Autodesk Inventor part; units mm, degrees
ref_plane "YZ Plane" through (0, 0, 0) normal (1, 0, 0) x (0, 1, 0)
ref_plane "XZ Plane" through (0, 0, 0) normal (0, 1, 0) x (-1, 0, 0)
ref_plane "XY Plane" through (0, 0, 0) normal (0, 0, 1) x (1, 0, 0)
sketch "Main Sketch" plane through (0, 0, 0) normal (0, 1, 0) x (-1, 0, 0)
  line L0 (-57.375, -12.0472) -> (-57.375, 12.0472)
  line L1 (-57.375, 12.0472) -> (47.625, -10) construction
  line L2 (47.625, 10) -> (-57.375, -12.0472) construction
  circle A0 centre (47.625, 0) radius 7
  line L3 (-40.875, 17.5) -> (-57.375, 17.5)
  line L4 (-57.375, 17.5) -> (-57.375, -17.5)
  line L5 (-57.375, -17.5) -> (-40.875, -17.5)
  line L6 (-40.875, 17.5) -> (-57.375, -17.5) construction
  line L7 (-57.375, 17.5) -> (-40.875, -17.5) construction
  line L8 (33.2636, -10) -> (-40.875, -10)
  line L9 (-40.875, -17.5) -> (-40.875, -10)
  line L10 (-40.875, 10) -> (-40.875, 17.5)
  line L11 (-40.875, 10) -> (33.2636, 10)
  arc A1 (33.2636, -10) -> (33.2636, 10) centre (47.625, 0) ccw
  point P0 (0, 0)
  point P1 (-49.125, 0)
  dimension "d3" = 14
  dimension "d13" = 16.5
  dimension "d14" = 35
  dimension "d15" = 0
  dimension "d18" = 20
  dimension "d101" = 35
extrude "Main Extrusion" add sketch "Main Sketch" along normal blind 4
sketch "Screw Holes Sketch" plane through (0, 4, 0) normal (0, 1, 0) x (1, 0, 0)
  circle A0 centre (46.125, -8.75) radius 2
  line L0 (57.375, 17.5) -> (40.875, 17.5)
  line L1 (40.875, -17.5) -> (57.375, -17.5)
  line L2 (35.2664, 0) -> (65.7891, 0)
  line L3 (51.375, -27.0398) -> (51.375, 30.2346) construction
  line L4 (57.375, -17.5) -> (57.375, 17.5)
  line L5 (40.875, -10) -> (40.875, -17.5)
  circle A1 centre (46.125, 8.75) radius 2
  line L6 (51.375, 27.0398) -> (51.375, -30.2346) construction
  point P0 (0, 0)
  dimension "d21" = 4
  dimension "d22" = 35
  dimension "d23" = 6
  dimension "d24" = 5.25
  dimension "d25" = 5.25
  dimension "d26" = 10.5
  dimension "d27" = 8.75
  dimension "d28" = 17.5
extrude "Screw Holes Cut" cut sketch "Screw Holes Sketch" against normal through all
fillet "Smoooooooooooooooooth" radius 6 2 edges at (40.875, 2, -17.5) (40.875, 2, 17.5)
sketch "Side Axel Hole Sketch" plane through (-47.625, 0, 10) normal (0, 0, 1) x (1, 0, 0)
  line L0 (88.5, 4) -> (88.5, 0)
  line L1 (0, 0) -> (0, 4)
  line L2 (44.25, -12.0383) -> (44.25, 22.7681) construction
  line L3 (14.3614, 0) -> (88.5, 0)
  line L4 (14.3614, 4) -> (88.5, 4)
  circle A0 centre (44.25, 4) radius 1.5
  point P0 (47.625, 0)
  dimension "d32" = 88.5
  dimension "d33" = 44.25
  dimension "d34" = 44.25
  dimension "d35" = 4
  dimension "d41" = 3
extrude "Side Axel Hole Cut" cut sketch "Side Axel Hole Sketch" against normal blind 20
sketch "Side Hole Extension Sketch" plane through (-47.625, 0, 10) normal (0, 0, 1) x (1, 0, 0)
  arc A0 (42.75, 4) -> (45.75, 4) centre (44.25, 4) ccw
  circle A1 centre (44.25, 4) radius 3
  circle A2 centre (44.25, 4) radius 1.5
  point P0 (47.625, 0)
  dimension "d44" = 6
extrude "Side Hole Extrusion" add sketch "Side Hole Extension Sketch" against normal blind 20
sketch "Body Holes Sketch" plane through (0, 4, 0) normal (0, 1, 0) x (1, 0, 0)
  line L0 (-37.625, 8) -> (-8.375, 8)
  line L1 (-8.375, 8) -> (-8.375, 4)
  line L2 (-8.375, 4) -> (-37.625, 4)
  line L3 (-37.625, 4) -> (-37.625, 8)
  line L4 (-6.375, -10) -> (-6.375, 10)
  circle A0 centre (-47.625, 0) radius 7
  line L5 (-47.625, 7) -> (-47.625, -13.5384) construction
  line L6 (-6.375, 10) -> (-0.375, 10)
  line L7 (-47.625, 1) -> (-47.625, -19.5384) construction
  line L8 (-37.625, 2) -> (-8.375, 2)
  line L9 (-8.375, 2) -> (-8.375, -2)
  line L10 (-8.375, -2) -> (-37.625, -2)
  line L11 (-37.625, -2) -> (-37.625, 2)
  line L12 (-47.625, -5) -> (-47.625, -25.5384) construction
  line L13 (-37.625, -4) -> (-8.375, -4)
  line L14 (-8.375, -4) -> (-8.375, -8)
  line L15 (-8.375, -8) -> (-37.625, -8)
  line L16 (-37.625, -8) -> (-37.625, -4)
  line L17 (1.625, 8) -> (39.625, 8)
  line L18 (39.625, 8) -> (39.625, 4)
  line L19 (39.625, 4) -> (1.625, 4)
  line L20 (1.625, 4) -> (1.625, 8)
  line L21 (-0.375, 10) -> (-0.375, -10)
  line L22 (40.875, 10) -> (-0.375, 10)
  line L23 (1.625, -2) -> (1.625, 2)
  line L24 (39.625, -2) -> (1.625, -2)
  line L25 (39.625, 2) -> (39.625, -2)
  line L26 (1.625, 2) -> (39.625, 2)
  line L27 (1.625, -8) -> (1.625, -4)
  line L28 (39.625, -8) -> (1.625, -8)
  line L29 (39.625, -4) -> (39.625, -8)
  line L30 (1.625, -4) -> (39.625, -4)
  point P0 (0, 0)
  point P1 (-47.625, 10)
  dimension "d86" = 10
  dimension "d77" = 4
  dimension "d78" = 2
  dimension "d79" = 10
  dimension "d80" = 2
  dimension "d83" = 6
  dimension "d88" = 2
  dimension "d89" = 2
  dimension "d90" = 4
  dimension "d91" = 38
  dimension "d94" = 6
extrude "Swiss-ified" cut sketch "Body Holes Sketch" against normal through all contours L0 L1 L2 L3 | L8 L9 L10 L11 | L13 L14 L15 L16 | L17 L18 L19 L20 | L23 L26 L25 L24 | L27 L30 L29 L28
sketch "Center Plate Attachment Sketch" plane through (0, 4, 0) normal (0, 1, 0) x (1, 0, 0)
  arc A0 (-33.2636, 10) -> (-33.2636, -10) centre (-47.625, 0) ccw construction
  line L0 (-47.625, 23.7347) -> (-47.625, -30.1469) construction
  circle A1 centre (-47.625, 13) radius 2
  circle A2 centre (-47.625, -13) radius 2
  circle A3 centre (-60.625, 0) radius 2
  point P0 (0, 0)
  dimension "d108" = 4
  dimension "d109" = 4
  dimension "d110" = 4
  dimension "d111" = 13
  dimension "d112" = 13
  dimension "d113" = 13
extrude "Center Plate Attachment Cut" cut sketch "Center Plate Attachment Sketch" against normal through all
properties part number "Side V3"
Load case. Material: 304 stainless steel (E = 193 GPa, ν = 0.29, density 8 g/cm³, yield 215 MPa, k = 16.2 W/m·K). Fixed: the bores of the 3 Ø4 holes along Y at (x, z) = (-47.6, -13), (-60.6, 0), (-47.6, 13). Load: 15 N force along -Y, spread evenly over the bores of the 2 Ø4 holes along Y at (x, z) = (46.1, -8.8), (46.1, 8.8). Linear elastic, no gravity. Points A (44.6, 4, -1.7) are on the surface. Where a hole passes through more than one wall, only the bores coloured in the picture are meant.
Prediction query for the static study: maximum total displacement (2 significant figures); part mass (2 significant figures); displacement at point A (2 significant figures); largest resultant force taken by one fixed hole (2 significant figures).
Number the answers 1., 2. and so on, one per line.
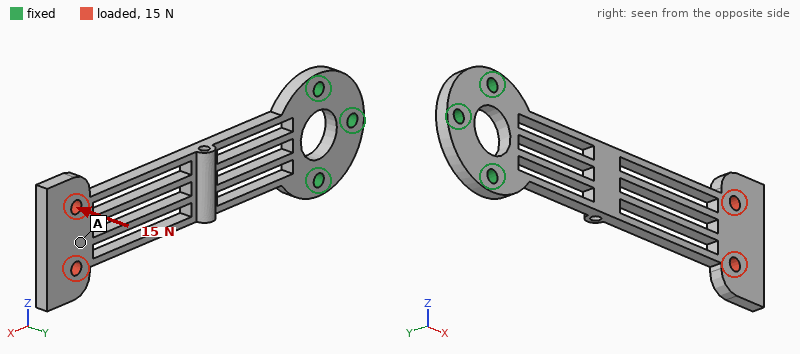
1. 0.46 mm
2. 63 g
3. 0.37 mm
4. 13 N
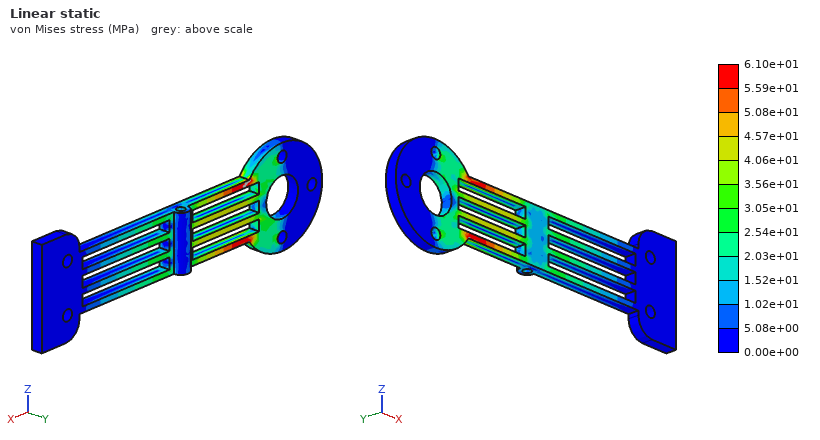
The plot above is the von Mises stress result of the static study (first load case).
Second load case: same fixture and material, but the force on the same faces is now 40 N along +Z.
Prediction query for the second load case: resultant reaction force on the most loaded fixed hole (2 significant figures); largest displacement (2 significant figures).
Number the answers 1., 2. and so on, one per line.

1. 160 N
2. 0.17 mm
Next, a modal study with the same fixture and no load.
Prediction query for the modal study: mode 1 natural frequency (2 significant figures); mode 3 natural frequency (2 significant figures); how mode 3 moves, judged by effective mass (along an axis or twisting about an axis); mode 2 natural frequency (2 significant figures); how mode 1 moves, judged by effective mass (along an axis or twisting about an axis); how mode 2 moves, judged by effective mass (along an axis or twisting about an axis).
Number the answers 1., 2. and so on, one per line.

1. 200 Hz
2. 900 Hz
3. twisting about X
4. 510 Hz
5. along Y
6. along Z
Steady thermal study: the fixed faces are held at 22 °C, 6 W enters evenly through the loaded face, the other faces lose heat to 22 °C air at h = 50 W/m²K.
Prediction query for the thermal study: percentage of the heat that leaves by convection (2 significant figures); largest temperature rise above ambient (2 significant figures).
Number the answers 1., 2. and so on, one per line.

1. 100 %
2. 66 K
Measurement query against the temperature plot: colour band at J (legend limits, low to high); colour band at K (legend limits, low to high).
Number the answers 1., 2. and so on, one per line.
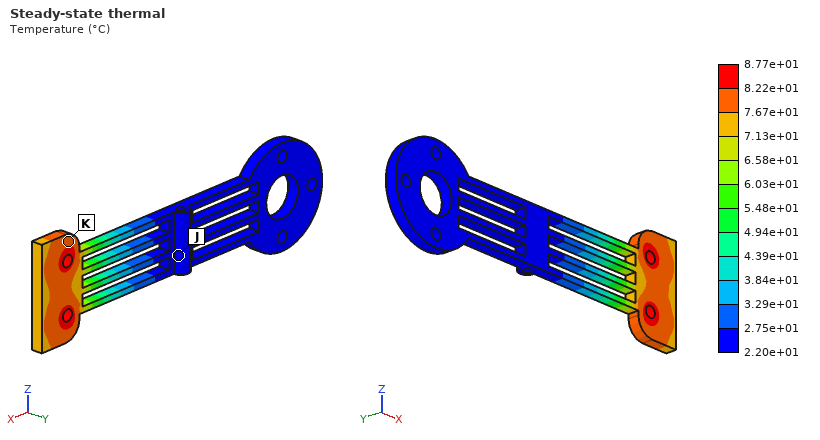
1. 2.20e+01 to 2.75e+01 °C
2. 7.67e+01 to 8.22e+01 °C
